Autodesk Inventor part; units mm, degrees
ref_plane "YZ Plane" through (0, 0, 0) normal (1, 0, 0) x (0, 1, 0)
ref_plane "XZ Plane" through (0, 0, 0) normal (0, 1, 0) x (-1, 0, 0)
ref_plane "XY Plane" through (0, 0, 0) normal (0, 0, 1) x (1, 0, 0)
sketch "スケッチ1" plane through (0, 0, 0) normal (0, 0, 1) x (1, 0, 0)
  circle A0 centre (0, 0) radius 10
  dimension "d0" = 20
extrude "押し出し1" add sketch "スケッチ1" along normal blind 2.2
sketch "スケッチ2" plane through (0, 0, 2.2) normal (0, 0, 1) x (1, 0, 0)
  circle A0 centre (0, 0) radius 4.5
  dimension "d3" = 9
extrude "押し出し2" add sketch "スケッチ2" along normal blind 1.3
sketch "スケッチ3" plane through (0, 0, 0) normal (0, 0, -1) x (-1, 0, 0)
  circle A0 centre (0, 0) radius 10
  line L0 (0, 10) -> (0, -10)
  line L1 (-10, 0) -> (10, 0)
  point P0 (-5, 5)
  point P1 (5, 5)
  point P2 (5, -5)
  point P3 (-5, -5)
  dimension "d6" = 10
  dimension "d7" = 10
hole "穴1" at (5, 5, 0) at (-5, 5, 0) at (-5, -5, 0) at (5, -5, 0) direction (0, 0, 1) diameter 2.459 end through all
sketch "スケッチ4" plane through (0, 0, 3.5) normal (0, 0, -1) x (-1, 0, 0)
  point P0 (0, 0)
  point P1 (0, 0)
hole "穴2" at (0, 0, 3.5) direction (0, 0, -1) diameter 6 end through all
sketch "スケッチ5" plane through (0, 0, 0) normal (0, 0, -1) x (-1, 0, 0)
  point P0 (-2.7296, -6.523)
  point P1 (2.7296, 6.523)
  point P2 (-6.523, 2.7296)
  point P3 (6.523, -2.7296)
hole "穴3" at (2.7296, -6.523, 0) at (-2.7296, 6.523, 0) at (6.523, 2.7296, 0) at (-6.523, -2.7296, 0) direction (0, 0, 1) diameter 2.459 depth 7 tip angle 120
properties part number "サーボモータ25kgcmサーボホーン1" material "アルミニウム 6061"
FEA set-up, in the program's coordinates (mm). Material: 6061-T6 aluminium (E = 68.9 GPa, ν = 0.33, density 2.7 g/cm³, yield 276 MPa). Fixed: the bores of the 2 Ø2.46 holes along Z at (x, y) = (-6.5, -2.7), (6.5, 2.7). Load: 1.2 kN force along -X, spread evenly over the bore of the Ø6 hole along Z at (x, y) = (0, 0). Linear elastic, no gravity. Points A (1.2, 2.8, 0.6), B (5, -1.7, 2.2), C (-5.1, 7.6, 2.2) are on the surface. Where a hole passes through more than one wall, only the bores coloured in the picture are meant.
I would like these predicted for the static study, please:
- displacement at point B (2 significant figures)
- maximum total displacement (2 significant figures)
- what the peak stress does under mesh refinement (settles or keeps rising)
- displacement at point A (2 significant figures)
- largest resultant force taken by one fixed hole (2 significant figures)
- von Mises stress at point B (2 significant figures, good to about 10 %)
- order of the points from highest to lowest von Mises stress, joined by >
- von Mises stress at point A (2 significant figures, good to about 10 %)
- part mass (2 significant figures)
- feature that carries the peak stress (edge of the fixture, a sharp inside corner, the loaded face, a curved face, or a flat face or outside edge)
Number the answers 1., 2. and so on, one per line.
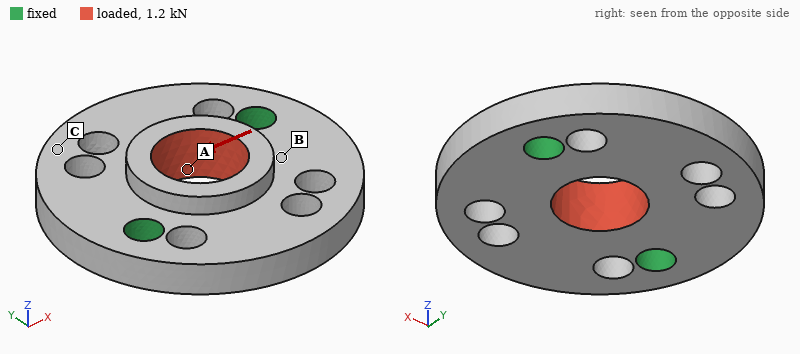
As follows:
1. 4.1 µm
2. 6.5 µm
3. keeps rising
4. 3.2 µm
5. 600 N
6. 32 MPa
7. A > B > C
8. 55 MPa
9. 1.6 g
10. edge of the fixture
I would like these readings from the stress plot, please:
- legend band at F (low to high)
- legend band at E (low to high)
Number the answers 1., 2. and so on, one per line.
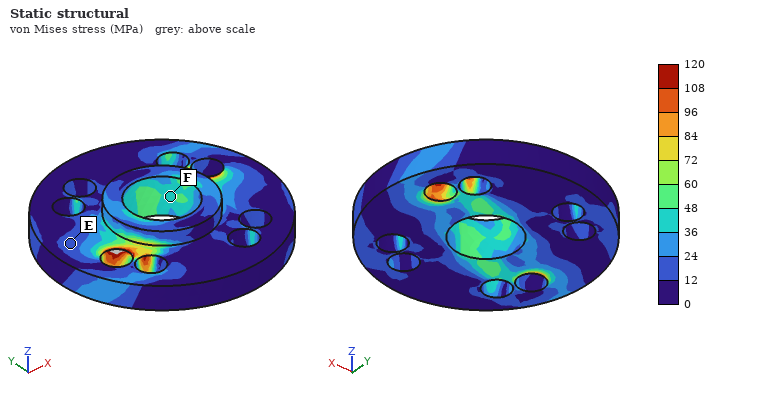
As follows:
1. 36 to 48 MPa
2. 12 to 24 MPa
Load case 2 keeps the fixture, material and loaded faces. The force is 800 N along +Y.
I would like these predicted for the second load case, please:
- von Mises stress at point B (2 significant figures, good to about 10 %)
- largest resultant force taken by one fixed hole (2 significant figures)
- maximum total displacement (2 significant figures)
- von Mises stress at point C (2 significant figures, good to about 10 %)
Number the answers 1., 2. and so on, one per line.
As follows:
1. 30 MPa
2. 400 N
3. 10 µm
4. 9.6 MPa
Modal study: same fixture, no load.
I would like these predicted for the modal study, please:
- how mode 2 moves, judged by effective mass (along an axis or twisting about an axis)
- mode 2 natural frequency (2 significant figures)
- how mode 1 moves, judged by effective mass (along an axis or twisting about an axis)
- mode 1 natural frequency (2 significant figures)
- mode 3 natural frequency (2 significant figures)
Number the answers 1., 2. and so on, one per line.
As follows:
1. along Z
2. 23 kHz
3. twisting about X
4. 18 kHz
5. 43 kHz
